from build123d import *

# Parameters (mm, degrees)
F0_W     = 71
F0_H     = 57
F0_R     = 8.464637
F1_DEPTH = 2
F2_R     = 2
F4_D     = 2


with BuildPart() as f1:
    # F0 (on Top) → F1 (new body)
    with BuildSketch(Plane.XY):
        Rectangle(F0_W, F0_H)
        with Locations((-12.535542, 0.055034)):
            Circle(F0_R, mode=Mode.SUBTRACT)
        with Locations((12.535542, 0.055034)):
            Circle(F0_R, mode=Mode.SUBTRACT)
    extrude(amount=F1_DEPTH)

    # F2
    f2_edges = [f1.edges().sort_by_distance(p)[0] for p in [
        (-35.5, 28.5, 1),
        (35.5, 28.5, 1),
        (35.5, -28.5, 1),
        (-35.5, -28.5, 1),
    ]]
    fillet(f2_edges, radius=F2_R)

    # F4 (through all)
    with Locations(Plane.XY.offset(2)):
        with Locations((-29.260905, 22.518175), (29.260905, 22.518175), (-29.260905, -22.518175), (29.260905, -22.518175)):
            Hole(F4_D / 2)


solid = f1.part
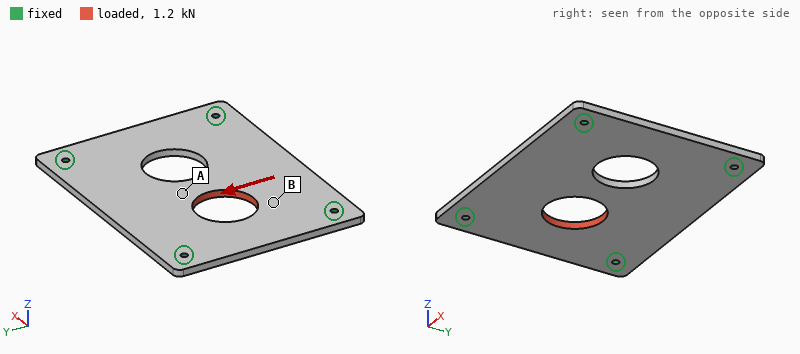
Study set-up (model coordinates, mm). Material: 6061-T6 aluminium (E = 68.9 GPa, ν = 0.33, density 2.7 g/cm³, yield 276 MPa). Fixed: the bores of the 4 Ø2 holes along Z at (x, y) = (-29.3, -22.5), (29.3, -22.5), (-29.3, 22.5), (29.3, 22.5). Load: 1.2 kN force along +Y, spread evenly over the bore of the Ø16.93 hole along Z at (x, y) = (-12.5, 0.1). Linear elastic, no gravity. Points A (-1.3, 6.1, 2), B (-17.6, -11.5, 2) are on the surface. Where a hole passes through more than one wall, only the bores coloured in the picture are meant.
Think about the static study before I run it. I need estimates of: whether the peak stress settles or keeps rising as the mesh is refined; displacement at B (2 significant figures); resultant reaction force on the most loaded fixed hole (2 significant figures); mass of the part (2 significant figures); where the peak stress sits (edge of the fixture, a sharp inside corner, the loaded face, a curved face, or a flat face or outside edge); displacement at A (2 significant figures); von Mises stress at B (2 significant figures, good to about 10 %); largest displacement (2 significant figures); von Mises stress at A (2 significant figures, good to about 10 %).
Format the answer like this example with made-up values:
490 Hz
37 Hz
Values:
keeps rising
6.4 µm
460 N
19 g
edge of the fixture
8.5 µm
14 MPa
9.7 µm
7.4 MPa
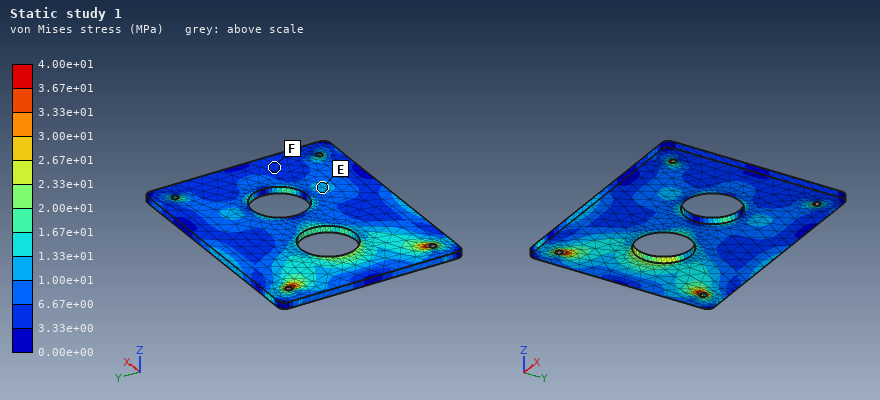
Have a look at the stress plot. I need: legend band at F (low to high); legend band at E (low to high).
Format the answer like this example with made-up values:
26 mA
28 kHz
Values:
3.33e+00 to 6.67e+00 MPa
1.00e+01 to 1.33e+01 MPa
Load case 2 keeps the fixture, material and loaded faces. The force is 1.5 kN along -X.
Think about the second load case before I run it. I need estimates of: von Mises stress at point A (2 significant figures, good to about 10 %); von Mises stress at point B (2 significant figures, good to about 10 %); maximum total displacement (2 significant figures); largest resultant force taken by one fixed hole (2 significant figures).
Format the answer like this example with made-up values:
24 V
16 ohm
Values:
19 MPa
15 MPa
11 µm
470 N
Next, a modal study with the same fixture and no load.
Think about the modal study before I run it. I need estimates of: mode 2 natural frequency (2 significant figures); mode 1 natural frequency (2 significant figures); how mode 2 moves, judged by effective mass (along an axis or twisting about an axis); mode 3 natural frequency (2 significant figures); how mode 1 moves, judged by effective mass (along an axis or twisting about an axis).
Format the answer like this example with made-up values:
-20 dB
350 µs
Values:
3400 Hz
2400 Hz
twisting about X
4500 Hz
along Z
